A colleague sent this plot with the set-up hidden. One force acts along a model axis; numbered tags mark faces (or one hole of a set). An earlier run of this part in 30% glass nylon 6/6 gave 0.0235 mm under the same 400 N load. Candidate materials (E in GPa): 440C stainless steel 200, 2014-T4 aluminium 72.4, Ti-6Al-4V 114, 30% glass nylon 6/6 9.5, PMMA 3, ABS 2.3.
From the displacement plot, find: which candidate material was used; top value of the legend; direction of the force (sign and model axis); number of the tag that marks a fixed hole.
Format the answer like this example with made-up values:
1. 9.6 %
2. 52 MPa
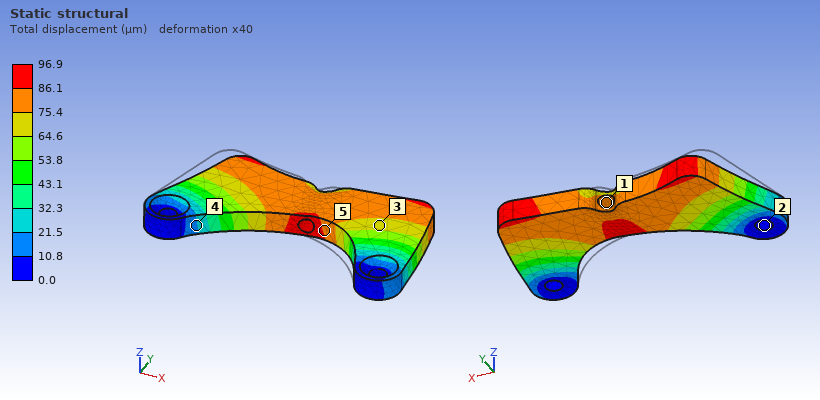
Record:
1. ABS
2. 96.9 µm
3. +X
4. 2
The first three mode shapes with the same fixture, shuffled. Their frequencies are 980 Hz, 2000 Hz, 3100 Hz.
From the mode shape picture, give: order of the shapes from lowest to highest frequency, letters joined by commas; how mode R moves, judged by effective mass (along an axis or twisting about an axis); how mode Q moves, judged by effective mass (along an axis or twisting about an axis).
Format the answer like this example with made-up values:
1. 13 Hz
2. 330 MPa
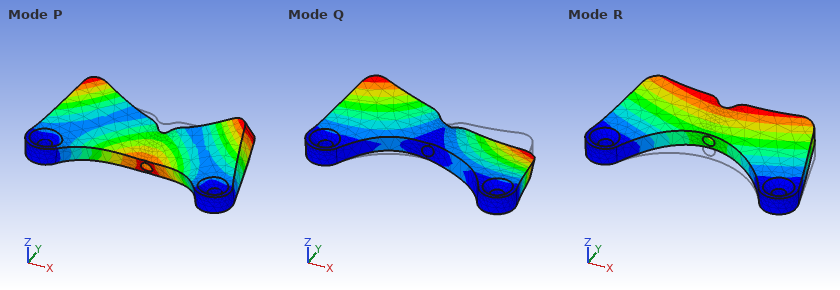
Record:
1. R, Q, P
2. along Z
3. twisting about Y
